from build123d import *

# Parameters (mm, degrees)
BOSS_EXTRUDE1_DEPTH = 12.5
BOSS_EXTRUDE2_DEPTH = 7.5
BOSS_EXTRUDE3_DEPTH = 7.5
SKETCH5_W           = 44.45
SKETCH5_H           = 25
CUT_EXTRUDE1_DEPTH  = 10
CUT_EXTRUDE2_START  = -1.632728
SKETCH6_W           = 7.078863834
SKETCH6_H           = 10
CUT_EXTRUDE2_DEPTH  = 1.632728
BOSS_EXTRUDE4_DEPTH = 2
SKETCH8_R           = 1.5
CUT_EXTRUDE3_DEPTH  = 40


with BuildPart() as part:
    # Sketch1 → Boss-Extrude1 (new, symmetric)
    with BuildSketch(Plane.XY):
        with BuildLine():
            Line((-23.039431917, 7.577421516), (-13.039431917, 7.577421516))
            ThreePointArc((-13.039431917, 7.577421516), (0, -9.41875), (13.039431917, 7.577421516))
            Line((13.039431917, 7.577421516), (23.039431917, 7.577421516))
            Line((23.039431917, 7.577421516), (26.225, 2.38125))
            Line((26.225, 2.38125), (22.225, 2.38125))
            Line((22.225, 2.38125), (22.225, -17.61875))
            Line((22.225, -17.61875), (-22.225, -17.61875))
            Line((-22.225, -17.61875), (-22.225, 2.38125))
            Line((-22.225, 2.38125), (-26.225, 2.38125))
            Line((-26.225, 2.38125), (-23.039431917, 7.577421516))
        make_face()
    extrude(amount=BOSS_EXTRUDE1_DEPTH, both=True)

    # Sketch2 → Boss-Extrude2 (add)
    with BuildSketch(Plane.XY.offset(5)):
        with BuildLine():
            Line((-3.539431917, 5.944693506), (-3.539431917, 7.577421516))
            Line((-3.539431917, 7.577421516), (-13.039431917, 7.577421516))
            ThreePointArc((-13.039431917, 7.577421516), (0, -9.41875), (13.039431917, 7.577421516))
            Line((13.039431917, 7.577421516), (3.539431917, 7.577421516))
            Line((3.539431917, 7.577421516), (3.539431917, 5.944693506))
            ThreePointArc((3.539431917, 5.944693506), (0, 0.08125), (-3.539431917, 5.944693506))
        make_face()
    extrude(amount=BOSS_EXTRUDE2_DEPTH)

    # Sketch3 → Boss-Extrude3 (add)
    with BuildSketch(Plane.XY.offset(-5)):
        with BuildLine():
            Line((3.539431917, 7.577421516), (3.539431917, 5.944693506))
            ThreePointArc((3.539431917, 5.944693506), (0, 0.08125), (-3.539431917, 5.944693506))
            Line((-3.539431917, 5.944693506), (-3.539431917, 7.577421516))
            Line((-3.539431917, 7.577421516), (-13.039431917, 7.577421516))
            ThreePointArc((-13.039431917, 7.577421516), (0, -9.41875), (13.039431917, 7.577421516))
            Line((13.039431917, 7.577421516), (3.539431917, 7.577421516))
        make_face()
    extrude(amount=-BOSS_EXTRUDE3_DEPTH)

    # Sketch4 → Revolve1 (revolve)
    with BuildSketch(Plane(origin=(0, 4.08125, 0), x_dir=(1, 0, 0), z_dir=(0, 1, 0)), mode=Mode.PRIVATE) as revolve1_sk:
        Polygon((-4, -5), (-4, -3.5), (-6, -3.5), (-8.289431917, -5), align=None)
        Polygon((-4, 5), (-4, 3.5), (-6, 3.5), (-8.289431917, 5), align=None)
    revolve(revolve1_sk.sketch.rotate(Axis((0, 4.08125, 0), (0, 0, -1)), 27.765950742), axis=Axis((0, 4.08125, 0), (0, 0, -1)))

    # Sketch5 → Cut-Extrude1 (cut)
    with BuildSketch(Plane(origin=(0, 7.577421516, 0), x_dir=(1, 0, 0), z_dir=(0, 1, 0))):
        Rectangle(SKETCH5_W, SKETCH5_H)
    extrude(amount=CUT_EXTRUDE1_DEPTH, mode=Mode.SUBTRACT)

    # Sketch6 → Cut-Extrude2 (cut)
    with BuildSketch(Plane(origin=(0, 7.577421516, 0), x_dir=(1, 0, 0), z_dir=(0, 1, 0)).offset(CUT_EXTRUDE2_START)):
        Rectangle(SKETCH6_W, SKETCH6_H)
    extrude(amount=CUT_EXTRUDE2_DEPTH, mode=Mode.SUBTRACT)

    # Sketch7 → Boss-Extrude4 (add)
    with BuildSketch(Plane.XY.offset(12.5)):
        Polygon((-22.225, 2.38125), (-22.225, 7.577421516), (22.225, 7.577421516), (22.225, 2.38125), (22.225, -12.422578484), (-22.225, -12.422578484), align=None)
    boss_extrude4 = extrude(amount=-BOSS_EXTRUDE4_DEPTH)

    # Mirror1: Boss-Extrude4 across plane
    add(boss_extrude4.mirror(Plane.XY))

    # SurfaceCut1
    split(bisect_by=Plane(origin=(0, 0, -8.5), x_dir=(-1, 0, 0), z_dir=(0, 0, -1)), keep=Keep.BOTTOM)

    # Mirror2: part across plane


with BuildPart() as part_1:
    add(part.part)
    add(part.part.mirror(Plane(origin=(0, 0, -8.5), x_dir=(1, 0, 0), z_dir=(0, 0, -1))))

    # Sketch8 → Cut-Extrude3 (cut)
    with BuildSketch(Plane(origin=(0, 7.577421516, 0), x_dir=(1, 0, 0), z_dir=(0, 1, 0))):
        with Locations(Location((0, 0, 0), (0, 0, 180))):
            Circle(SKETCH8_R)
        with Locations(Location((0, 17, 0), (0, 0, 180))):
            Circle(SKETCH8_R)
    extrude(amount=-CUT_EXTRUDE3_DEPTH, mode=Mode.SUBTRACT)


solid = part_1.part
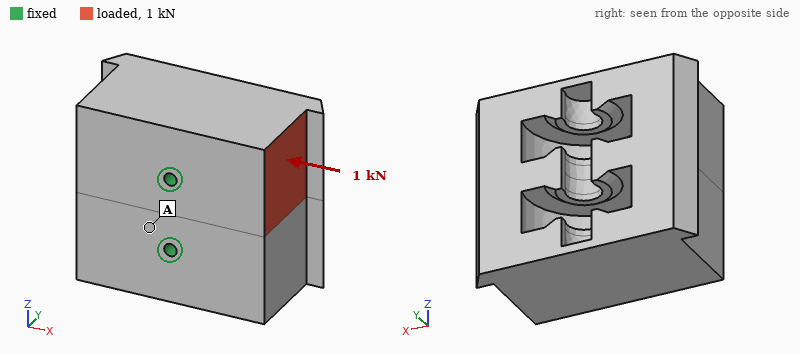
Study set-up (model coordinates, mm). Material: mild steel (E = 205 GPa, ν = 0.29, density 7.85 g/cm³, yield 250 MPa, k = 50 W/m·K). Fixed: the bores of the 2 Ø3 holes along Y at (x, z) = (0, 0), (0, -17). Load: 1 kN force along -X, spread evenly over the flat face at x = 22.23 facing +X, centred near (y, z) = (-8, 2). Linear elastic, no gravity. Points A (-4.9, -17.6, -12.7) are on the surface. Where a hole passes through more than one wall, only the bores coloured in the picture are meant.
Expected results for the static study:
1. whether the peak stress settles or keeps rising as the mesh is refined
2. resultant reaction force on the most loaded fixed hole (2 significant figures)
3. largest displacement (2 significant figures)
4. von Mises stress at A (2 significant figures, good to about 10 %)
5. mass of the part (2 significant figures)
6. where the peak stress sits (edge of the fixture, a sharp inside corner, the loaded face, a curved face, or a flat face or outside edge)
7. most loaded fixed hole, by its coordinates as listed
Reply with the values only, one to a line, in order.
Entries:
keeps rising
1.1 kN
3.3 µm
3.7 MPa
310 g
edge of the fixture
(0, 0)
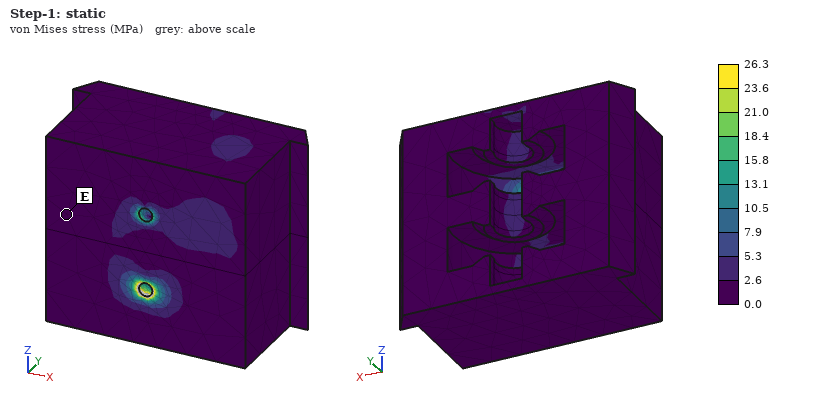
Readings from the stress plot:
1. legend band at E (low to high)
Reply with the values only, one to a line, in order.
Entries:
0.0 to 2.6 MPa
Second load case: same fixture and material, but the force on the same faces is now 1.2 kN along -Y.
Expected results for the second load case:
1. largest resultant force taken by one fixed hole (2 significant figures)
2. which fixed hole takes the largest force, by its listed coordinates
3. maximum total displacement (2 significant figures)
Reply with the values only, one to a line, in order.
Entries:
1.2 kN
(0, 0)
15 µm
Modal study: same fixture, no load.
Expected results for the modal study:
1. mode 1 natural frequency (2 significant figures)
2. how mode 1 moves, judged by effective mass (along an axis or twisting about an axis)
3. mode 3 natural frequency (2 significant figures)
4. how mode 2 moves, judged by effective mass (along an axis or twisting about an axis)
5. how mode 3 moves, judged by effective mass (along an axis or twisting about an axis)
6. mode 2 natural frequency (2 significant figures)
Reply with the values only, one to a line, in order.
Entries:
4400 Hz
along X
9800 Hz
along Z
twisting about Y
8500 Hz
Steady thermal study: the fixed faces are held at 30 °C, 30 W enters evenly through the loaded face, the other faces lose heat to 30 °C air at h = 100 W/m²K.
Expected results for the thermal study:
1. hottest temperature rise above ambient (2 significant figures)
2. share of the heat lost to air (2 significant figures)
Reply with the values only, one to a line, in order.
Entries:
31 K
31 %
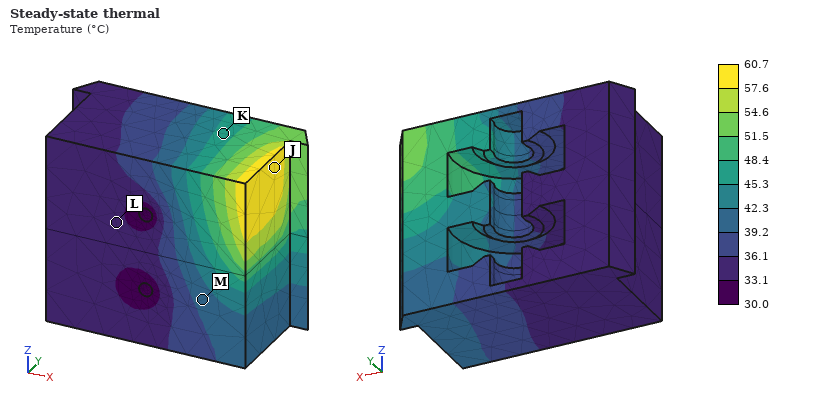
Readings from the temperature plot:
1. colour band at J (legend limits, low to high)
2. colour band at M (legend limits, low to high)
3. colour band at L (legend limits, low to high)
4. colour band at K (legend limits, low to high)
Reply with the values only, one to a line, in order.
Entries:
57.6 to 60.7 °C
39.2 to 42.3 °C
33.1 to 36.1 °C
45.3 to 48.4 °C
